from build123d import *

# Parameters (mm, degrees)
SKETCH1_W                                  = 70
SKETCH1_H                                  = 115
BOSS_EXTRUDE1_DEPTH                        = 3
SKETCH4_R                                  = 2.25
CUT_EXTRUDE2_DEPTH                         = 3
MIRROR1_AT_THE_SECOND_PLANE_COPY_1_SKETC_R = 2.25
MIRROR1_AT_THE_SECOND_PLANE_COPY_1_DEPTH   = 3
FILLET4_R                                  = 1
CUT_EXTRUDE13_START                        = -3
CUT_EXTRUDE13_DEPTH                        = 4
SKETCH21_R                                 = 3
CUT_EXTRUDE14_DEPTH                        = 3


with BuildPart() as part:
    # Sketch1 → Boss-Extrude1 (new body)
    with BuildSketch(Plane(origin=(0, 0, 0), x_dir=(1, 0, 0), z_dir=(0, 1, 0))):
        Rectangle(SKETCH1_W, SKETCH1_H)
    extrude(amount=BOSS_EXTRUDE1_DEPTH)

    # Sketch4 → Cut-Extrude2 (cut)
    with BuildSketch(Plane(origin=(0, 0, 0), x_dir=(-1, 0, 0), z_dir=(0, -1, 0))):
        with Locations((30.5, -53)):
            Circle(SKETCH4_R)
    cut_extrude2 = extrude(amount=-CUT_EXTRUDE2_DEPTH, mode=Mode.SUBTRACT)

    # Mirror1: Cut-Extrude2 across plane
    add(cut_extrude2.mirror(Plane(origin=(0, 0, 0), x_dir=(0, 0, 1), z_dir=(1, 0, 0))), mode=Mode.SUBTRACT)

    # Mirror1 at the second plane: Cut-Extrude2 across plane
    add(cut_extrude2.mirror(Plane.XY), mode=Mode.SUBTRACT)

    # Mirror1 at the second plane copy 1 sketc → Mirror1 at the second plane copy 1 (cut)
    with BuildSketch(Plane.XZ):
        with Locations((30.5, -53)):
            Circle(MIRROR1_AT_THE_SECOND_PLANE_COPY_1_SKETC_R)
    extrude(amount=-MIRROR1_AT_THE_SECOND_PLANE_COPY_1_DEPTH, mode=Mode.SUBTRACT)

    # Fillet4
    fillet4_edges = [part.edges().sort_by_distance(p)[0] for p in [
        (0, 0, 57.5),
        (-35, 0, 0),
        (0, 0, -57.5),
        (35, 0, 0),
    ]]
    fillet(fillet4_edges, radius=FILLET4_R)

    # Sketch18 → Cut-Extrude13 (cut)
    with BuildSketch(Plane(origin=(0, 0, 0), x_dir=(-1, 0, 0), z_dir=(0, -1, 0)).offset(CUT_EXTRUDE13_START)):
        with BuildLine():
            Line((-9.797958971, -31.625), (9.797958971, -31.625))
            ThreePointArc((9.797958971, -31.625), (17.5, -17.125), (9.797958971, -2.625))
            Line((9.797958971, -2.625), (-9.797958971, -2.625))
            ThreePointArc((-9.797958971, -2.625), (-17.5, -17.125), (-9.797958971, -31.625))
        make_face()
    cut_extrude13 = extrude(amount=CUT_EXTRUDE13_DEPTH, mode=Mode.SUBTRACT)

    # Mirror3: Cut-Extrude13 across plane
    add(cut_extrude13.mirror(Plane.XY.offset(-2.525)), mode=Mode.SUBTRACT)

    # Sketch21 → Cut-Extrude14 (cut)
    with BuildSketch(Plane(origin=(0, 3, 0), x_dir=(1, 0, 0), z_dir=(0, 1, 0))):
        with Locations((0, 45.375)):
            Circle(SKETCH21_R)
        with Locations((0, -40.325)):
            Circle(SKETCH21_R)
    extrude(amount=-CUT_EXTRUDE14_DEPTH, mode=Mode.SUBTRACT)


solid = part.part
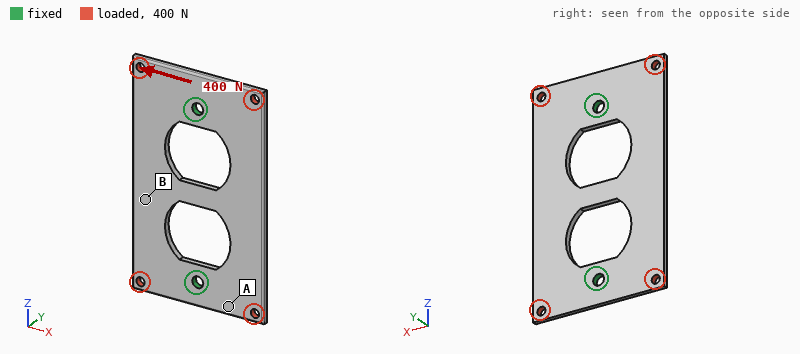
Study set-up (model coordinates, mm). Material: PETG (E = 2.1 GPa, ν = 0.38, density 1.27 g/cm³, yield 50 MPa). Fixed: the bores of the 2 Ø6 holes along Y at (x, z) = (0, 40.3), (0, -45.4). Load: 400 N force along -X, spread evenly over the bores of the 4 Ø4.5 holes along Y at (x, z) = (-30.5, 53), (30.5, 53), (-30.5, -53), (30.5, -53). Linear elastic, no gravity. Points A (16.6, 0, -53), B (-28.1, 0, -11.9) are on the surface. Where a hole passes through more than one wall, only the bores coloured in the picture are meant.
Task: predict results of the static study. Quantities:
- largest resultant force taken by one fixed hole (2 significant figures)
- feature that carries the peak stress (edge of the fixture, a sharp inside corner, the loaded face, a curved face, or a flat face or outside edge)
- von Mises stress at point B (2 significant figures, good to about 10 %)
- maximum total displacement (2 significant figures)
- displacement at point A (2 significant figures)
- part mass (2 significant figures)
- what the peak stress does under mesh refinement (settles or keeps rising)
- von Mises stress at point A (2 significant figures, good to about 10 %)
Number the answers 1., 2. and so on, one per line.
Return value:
1. 210 N
2. edge of the fixture
3. 0.78 MPa
4. 83 µm
5. 22 µm
6. 23 g
7. keeps rising
8. 2.5 MPa
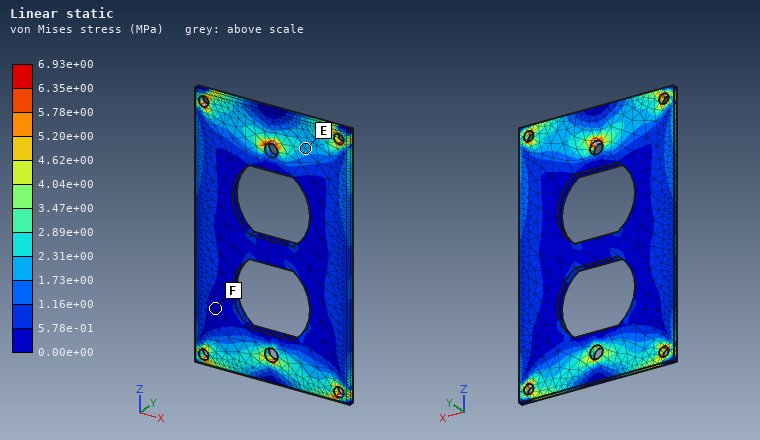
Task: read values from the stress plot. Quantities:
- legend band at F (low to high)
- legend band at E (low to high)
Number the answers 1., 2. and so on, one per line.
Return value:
1. 0.00e+00 to 5.78e-01 MPa
2. 1.73e+00 to 2.31e+00 MPa
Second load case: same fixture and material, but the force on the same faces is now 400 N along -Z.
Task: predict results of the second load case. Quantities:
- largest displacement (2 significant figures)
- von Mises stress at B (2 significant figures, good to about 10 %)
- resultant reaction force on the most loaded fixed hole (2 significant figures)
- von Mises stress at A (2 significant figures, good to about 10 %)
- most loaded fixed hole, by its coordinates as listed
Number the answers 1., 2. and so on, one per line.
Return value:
1. 0.15 mm
2. 1.3 MPa
3. 220 N
4. 1.6 MPa
5. (0, 40.3)
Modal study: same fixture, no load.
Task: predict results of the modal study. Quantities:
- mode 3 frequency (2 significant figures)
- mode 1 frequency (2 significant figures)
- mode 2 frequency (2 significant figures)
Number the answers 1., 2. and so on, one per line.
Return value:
1. 570 Hz
2. 310 Hz
3. 310 Hz
